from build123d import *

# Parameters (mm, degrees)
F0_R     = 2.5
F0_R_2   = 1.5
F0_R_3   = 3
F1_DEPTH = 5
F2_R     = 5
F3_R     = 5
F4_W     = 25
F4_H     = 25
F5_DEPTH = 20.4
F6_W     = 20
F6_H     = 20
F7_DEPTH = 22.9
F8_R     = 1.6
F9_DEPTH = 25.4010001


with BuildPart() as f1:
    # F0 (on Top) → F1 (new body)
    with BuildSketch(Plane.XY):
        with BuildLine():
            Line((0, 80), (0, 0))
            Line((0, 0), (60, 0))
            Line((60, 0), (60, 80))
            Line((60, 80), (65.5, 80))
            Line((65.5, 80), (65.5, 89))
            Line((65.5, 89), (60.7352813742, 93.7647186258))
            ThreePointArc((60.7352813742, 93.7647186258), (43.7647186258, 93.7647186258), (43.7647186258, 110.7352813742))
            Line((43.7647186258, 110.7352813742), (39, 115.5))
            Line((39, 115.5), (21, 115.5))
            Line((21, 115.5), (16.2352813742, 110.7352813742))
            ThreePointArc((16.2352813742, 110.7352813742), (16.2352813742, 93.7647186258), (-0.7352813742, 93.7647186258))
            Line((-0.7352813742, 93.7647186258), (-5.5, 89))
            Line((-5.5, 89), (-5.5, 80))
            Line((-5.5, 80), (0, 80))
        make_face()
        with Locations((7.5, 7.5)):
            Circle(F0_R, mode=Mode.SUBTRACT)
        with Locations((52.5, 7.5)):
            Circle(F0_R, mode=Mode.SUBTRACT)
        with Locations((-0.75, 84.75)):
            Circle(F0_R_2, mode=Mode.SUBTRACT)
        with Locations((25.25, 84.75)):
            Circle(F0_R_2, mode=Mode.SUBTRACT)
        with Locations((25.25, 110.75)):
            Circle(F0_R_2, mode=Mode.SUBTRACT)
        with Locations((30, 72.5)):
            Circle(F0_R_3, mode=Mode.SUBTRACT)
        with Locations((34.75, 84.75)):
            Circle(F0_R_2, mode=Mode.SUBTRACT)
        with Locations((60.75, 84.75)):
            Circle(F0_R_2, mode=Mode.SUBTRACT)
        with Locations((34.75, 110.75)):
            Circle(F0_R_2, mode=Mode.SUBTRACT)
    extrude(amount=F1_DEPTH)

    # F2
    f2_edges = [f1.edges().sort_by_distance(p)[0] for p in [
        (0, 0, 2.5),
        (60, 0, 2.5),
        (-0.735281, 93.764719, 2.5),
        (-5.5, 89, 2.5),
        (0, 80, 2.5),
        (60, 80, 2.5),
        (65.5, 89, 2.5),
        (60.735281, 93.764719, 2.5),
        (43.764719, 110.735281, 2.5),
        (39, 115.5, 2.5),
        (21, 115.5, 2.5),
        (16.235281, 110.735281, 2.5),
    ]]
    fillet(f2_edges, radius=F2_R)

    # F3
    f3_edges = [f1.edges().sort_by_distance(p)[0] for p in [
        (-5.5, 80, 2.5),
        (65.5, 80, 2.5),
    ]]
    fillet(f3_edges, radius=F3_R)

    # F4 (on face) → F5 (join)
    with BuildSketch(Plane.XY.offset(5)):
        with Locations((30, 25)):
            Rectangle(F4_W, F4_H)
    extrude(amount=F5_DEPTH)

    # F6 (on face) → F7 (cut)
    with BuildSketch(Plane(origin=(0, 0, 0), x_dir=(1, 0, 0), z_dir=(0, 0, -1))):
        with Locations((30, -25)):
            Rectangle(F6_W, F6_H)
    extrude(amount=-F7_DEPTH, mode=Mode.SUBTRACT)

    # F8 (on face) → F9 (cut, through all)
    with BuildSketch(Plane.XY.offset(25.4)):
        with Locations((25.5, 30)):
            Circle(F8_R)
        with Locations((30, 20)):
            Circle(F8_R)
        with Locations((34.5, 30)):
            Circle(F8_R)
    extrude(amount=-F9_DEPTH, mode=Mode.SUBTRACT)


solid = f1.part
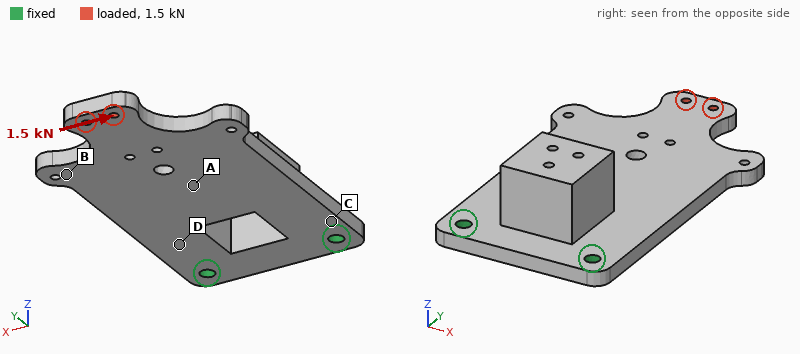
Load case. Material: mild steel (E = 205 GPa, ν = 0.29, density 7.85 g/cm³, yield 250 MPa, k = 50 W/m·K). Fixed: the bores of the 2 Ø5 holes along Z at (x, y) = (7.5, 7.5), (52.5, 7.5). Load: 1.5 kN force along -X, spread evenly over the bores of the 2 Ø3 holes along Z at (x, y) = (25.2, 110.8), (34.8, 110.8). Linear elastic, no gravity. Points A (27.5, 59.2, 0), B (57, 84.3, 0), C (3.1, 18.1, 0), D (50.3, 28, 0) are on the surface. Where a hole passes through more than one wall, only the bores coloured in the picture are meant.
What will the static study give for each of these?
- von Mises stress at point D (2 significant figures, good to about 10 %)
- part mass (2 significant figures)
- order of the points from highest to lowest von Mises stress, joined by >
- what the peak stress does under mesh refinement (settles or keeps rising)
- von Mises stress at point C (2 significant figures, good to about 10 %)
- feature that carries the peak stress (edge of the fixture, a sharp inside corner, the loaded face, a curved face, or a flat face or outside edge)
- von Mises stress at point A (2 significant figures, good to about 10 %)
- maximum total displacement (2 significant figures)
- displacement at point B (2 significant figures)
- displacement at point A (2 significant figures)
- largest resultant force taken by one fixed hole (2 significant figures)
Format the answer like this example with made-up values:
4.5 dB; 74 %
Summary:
36 MPa; 260 g; C > D > A > B; keeps rising; 44 MPa; edge of the fixture; 15 MPa; 55 µm; 32 µm; 18 µm; 3.3 kN
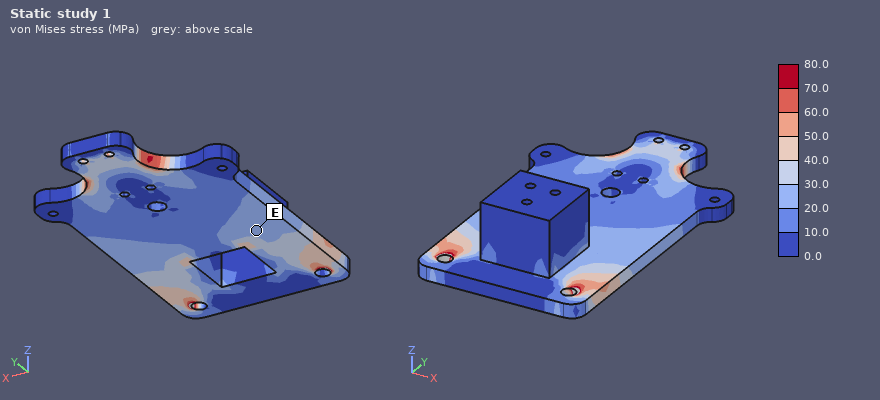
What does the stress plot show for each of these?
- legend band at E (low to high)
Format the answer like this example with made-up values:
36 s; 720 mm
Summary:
20.0 to 30.0 MPa
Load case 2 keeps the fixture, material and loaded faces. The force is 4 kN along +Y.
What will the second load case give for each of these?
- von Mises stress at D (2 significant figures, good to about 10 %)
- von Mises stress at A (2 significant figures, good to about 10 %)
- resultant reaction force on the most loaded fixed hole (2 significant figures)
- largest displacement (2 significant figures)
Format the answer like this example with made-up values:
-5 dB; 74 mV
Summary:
22 MPa; 12 MPa; 2.0 kN; 18 µm
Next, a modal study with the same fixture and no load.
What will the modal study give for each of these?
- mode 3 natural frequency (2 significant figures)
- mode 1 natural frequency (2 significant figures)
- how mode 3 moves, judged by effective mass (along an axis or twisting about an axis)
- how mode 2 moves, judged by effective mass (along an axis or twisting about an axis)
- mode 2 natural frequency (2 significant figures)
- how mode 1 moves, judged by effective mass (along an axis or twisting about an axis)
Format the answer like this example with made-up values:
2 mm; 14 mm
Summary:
2300 Hz; 470 Hz; along Z; twisting about Y; 2000 Hz; along Z
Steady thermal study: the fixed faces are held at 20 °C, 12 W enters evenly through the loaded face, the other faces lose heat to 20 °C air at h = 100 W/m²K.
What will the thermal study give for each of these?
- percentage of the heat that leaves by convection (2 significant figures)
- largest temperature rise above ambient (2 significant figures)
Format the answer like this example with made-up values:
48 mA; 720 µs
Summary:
94 %; 52 K
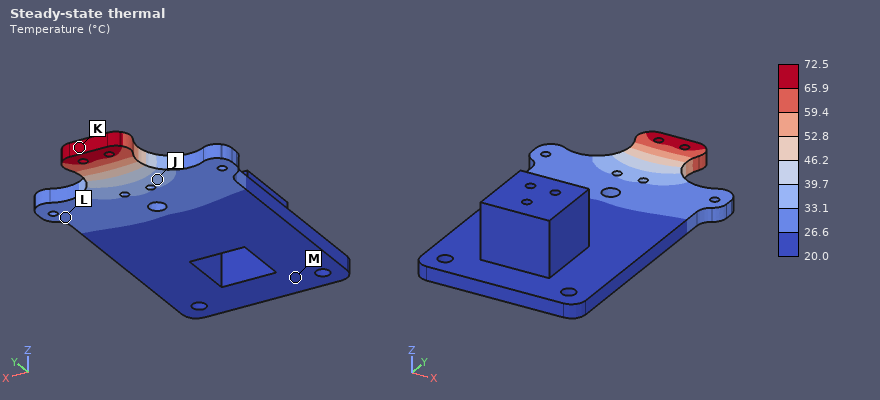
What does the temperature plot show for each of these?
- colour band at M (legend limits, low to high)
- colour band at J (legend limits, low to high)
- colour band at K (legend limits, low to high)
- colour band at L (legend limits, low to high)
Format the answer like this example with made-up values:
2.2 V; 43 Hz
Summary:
20.0 to 26.6 °C; 33.1 to 39.7 °C; 65.9 to 72.5 °C; 26.6 to 33.1 °C
